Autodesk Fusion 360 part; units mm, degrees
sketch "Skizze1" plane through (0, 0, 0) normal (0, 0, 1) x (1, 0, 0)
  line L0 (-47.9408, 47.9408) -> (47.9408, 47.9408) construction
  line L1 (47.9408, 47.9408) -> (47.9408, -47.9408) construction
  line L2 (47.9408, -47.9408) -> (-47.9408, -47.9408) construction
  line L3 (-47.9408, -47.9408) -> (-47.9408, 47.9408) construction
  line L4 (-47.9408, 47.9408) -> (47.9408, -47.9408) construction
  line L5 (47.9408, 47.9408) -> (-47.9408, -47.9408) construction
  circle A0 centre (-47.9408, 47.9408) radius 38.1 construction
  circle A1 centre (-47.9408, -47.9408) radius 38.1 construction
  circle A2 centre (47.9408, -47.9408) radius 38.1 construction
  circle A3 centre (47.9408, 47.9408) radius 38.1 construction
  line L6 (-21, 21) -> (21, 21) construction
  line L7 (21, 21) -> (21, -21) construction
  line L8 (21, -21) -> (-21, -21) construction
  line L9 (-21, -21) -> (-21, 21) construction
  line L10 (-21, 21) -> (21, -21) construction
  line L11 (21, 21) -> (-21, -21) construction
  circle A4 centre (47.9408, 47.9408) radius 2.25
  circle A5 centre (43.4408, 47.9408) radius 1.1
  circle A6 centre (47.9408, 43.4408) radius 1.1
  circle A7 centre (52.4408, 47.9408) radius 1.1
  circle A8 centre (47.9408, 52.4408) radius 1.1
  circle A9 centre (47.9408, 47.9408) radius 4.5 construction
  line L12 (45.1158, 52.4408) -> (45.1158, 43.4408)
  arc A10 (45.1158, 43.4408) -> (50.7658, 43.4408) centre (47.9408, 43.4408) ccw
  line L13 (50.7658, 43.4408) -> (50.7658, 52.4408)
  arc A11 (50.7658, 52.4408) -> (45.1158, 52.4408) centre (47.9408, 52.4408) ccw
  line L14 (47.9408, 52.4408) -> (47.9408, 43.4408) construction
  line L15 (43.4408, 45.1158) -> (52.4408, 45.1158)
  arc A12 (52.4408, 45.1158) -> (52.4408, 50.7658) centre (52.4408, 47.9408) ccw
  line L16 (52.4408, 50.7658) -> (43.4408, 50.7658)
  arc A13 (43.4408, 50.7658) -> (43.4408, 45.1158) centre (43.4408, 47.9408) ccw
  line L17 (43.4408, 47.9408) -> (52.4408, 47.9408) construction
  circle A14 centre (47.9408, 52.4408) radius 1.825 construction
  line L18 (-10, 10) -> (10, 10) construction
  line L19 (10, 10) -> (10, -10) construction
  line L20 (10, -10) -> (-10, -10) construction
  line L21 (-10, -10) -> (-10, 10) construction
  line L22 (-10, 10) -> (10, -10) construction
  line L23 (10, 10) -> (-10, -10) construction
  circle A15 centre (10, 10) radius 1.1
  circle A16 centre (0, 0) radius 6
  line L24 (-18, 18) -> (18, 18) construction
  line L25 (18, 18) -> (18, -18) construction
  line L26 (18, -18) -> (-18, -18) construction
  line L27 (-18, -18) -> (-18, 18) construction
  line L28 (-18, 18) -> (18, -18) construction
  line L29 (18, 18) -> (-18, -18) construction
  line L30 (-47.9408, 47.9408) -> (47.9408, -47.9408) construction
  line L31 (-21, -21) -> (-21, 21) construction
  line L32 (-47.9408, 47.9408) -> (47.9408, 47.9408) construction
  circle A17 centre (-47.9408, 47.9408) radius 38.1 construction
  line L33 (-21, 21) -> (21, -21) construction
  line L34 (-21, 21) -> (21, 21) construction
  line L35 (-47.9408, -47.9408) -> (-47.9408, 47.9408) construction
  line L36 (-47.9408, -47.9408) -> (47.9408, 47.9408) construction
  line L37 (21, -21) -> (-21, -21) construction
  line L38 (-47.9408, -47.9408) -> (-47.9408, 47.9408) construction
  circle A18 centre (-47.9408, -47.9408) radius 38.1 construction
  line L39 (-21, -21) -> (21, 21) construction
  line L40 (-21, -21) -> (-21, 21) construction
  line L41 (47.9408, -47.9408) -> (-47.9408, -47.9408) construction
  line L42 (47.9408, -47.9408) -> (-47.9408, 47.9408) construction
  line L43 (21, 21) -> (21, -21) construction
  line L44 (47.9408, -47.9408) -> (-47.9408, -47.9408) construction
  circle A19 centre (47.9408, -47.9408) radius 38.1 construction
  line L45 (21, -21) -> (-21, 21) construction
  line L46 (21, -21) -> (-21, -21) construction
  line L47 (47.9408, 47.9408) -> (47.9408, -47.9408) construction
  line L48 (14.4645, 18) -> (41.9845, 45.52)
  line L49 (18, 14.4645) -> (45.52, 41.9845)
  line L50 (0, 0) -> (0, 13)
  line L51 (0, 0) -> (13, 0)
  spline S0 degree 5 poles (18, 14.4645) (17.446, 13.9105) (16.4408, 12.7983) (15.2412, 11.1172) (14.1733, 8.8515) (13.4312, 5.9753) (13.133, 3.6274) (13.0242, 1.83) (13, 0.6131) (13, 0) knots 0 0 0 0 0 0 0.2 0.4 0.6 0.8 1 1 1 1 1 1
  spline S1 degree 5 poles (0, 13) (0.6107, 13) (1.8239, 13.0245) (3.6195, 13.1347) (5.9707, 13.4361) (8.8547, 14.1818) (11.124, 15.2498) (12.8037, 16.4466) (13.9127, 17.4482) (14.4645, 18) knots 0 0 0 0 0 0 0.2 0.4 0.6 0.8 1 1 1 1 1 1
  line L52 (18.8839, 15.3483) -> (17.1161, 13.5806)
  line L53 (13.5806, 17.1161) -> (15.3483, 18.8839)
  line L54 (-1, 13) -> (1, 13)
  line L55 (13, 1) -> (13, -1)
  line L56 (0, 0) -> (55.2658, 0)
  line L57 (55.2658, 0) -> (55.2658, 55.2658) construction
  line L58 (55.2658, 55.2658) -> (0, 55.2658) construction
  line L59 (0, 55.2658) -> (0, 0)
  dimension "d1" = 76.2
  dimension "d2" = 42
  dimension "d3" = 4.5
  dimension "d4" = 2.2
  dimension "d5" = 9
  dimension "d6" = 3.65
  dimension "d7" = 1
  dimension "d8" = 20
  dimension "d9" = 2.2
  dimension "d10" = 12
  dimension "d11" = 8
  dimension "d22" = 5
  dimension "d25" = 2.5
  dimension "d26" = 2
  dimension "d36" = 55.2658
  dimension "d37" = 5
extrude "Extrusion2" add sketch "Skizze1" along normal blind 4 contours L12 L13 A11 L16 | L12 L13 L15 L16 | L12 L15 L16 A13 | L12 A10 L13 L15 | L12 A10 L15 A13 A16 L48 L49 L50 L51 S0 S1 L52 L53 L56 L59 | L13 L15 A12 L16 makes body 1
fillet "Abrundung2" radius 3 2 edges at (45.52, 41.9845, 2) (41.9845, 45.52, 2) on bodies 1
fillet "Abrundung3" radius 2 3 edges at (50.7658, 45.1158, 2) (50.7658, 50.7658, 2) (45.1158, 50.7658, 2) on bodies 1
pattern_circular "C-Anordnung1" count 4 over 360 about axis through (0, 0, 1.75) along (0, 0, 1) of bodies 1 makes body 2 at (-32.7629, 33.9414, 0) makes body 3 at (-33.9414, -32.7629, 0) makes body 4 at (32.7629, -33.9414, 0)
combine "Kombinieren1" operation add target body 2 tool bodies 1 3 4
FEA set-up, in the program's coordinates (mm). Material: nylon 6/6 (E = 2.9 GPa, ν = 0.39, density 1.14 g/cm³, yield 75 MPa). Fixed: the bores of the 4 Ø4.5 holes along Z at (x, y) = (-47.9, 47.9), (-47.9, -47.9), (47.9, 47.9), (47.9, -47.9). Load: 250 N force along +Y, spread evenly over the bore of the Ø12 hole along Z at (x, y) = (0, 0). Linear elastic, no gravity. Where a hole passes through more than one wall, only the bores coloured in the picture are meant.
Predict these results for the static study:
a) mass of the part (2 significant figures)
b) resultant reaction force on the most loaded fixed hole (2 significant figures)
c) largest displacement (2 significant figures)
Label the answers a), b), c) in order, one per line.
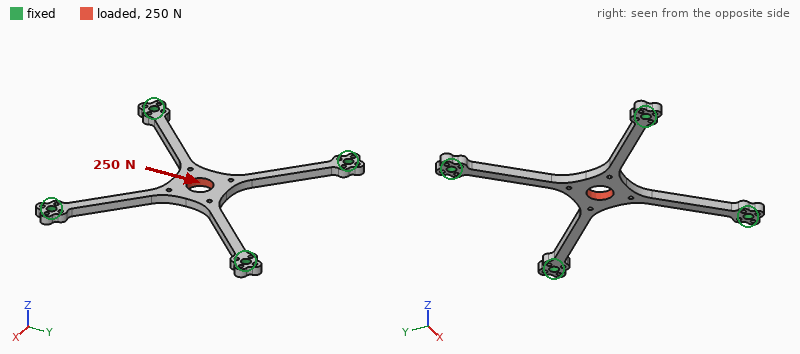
a) 8.6 g
b) 87 N
c) 0.12 mm
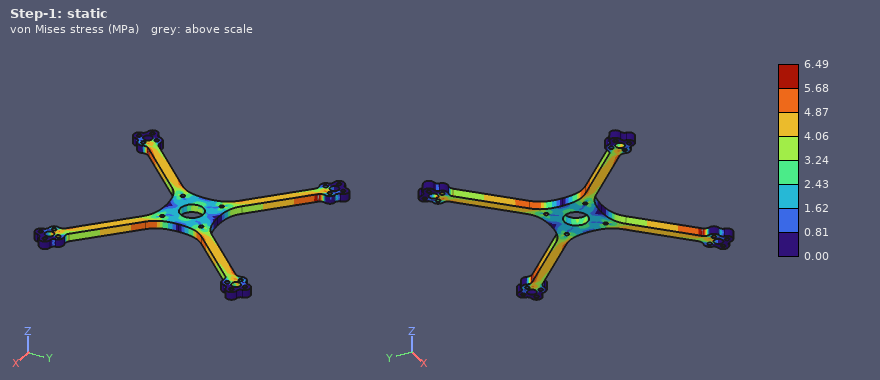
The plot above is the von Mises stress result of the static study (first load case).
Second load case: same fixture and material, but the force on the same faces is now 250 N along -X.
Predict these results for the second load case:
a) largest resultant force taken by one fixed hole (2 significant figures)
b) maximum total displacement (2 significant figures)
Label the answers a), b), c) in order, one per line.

a) 87 N
b) 0.12 mm
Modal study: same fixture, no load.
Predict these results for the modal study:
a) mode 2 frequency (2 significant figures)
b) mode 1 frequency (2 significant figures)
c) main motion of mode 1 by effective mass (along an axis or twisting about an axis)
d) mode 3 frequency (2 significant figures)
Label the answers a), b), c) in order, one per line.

a) 1000 Hz
b) 370 Hz
c) along Z
d) 1000 Hz
